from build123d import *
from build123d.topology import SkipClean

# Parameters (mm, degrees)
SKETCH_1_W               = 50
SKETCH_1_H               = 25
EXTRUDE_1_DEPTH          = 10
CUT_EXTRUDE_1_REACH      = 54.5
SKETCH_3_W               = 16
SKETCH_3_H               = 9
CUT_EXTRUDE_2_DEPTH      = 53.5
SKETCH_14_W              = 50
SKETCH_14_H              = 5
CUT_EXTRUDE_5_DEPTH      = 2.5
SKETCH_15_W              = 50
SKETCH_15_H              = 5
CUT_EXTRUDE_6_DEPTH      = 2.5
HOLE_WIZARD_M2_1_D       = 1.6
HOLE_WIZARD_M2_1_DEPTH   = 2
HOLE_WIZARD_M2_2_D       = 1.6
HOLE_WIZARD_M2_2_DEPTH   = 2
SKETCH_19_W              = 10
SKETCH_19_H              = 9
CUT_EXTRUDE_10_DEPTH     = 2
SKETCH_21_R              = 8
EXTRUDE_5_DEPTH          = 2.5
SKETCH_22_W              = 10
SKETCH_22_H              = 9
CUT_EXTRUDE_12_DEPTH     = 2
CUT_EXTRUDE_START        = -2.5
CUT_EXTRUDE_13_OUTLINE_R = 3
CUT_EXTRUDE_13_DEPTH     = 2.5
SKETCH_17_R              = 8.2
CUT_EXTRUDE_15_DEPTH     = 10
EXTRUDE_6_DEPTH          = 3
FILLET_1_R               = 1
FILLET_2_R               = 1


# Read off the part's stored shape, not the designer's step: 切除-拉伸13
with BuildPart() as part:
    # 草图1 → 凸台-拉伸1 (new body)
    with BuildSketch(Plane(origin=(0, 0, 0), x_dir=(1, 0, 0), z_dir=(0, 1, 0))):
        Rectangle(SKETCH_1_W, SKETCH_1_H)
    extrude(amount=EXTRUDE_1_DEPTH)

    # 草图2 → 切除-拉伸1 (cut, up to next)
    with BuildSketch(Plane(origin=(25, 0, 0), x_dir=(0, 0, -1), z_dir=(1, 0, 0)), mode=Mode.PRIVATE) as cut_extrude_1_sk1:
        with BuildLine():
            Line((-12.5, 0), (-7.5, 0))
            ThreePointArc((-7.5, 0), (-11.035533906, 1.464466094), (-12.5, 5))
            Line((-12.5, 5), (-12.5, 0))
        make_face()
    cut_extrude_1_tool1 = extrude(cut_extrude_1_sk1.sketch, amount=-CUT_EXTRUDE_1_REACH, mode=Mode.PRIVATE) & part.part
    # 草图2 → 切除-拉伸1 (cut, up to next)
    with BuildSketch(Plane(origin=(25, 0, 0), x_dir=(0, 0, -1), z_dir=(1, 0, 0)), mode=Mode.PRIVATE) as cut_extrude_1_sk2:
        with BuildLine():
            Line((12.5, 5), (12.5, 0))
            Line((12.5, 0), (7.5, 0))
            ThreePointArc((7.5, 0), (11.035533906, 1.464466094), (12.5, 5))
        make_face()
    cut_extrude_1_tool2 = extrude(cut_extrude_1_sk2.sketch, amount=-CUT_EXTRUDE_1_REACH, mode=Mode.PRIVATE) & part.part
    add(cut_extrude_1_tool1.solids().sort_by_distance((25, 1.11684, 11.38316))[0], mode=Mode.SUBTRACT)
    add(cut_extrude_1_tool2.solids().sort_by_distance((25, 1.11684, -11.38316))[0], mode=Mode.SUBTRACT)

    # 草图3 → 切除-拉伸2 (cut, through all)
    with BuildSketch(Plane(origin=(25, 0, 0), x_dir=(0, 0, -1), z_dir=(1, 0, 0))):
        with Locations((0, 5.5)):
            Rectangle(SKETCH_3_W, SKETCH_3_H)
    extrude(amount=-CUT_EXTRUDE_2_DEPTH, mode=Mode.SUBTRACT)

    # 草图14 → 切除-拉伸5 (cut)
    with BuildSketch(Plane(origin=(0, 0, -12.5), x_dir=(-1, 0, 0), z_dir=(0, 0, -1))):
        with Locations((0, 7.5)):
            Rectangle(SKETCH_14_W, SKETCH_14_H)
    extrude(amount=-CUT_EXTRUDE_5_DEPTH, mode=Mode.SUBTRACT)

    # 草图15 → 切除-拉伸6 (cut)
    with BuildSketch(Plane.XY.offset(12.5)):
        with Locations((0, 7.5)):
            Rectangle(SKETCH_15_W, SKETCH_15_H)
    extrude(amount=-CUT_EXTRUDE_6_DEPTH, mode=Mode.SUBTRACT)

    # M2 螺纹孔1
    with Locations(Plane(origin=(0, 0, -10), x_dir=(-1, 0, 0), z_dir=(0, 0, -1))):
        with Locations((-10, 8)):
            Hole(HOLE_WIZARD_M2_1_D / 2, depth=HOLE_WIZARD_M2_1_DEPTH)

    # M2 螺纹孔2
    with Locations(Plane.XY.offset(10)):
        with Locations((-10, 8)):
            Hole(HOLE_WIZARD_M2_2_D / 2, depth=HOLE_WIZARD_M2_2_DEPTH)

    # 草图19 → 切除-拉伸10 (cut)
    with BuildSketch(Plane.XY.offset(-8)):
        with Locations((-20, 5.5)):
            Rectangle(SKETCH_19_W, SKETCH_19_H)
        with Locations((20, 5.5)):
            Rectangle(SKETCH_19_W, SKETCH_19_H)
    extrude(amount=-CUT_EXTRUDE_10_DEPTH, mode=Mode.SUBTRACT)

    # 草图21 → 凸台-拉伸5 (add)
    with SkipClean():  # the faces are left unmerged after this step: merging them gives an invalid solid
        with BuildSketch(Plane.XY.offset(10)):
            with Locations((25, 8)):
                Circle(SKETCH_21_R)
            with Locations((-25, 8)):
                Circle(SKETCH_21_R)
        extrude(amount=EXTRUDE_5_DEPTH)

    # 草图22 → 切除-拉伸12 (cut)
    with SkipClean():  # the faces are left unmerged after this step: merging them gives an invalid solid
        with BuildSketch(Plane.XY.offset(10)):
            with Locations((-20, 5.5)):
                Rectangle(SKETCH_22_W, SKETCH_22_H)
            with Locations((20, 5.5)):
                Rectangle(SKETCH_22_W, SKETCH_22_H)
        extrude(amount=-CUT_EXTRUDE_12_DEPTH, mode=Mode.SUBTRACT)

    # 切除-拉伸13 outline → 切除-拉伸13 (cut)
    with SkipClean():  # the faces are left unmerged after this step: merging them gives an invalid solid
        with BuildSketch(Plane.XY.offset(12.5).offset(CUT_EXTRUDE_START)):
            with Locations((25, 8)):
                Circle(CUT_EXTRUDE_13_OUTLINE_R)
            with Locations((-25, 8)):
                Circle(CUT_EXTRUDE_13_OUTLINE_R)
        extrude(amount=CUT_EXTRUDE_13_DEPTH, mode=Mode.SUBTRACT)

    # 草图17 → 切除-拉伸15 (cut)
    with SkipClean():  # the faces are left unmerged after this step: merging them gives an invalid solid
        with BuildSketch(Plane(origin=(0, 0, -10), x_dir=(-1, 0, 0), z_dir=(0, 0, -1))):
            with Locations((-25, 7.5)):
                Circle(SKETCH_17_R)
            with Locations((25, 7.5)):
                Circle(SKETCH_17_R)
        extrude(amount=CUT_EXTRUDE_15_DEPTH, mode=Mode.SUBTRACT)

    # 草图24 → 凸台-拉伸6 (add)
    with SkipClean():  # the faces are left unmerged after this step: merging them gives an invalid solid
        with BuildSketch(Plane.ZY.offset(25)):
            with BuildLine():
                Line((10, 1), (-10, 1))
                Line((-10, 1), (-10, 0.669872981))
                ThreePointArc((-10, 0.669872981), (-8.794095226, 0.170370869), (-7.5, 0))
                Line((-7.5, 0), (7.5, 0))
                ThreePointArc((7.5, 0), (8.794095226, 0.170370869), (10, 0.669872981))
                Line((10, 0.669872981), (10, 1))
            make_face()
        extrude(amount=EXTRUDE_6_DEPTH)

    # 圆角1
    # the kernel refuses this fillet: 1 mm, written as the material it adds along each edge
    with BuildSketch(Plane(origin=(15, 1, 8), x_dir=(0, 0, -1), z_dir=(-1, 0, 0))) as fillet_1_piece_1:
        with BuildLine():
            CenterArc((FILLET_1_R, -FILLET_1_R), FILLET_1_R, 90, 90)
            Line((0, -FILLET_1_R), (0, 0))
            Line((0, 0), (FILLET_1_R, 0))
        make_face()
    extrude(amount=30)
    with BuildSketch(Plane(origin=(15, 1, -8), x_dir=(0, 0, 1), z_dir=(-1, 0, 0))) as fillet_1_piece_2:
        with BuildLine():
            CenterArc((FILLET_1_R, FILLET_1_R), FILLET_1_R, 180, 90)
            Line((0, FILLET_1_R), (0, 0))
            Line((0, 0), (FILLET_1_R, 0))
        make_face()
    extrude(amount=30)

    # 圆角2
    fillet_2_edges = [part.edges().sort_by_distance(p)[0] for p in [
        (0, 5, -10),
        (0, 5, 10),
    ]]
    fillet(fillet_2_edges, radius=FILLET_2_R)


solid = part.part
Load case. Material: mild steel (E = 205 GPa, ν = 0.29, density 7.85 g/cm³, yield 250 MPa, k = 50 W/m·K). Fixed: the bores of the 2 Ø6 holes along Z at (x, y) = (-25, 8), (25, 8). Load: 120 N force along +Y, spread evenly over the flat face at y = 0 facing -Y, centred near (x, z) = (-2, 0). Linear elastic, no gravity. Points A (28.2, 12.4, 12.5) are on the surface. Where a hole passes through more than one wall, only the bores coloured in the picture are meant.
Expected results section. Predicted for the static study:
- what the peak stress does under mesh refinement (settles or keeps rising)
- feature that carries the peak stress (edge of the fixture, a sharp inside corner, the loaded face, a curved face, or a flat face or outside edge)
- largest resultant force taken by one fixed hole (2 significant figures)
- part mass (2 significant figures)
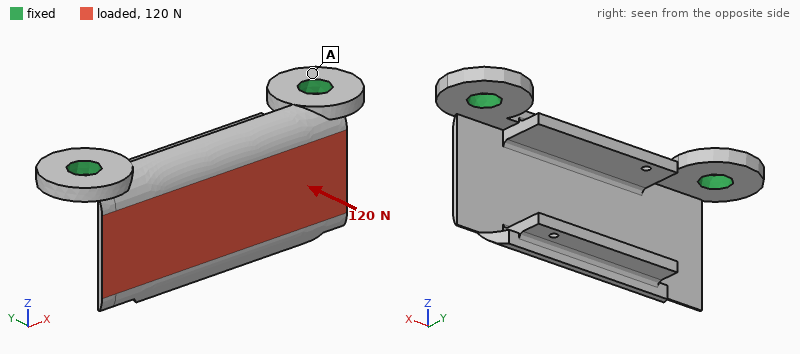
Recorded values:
keeps rising
a sharp inside corner
72 N
28 g
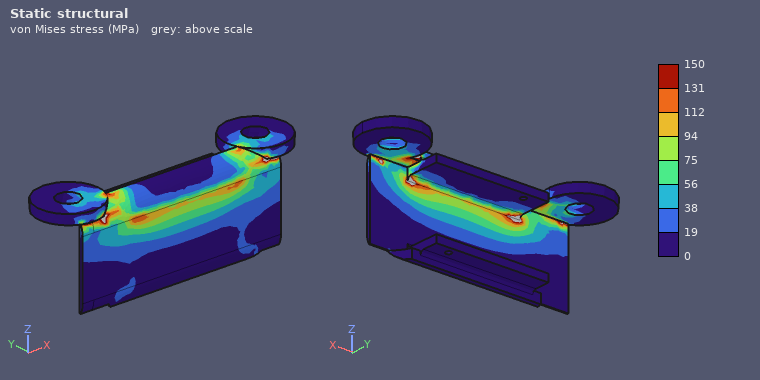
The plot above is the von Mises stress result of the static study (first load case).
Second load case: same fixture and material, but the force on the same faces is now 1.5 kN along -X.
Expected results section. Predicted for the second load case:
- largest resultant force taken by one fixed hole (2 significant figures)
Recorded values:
850 N
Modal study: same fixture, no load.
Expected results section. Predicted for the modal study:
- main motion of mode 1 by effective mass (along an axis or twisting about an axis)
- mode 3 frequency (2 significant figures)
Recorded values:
along Y
4200 Hz
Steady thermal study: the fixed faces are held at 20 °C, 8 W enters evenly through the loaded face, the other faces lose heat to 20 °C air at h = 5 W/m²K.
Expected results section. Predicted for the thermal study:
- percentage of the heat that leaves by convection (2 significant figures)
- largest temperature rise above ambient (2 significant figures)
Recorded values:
9.2 %
61 K
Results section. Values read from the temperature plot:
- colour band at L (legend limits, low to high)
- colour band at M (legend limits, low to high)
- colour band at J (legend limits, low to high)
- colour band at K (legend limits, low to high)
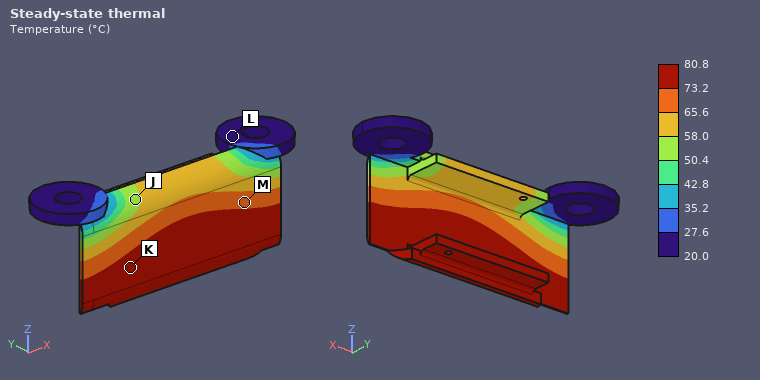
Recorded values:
20.0 to 27.6 °C
65.6 to 73.2 °C
50.4 to 58.0 °C
73.2 to 80.8 °C
